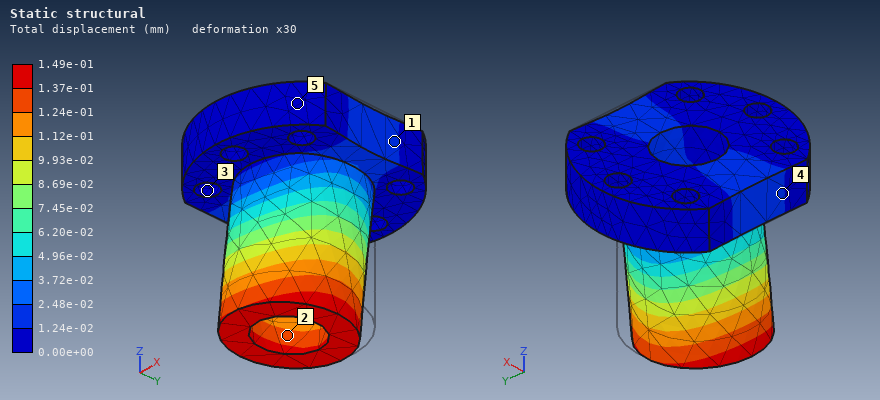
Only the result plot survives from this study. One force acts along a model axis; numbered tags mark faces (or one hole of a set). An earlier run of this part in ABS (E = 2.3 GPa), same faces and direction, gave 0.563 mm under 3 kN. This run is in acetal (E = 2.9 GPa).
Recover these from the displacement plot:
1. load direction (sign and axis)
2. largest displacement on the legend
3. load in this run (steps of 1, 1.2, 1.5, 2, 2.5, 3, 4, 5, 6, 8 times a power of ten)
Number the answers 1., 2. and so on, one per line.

1. -X
2. 1.49e-01 mm
3. 1 kN
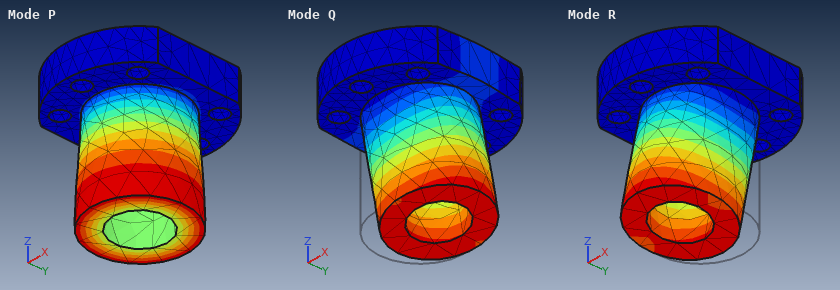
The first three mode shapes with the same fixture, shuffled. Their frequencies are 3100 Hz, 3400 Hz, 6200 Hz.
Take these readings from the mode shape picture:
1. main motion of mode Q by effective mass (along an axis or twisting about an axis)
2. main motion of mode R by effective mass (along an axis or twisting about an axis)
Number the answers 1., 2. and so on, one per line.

1. along X
2. along Y
